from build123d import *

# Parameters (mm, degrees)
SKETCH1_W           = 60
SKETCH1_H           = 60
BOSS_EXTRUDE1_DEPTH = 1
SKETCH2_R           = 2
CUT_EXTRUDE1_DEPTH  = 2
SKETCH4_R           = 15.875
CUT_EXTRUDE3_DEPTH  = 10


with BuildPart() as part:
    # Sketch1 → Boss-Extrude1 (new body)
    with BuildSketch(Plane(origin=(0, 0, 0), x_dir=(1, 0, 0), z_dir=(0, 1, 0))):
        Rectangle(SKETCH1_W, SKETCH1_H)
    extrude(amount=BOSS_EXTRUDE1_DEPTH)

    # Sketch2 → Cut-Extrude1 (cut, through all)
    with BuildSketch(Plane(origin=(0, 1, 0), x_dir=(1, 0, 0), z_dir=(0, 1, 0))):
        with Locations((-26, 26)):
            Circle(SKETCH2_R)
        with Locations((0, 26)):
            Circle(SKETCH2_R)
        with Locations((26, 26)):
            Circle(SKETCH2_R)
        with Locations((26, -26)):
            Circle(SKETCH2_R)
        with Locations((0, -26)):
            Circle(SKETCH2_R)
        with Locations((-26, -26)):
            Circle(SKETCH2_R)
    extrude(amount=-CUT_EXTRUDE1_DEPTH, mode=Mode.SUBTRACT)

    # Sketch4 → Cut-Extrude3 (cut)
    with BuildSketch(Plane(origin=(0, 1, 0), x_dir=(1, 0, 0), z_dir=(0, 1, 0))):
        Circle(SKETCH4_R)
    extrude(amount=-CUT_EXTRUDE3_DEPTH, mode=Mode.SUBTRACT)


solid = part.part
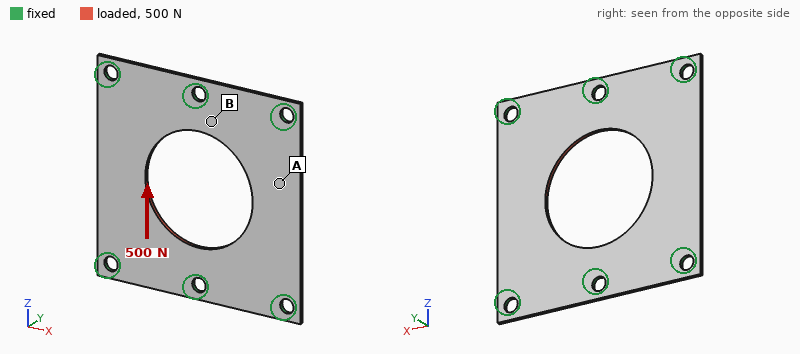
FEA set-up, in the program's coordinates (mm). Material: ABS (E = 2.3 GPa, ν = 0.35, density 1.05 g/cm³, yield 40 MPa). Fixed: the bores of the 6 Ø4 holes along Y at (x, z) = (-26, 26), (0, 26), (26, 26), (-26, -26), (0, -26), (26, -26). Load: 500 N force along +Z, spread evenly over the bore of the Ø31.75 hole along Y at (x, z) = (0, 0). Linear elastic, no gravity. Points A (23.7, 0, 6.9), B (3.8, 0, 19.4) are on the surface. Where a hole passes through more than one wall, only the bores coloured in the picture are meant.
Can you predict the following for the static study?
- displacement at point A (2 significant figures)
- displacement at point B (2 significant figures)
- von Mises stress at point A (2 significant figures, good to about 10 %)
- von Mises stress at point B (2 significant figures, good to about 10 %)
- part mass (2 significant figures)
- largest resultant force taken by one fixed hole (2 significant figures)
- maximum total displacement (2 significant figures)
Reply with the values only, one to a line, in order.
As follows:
33 µm
29 µm
2.5 MPa
7.5 MPa
2.9 g
120 N
64 µm
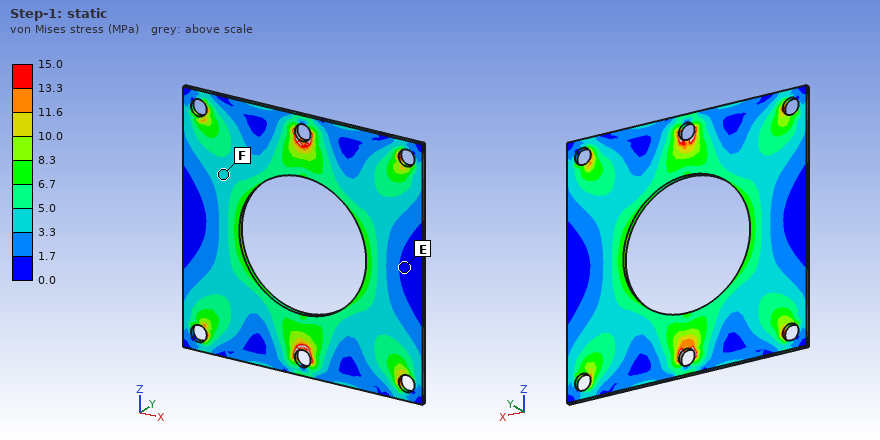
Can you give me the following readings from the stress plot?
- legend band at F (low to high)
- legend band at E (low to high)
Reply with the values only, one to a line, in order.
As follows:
3.3 to 5.0 MPa
0.0 to 1.7 MPa
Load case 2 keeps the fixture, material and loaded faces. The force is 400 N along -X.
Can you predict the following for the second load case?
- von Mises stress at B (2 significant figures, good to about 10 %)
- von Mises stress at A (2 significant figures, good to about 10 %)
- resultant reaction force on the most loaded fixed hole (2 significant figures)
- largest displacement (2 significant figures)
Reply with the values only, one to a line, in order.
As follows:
8.8 MPa
4.1 MPa
100 N
0.12 mm
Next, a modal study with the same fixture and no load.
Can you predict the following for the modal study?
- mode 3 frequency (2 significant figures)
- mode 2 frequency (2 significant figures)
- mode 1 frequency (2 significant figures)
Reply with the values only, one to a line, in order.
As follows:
1400 Hz
660 Hz
660 Hz
